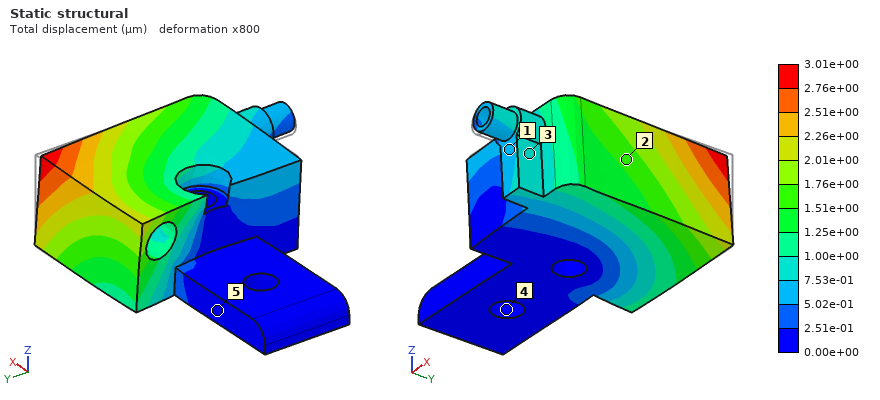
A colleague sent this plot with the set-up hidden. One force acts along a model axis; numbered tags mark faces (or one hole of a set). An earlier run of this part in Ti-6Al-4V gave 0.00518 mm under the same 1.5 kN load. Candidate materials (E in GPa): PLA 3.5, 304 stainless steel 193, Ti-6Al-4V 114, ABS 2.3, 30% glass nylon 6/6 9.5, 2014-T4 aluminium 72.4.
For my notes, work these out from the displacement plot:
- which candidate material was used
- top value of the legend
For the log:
304 stainless steel
3.01e+00 µm
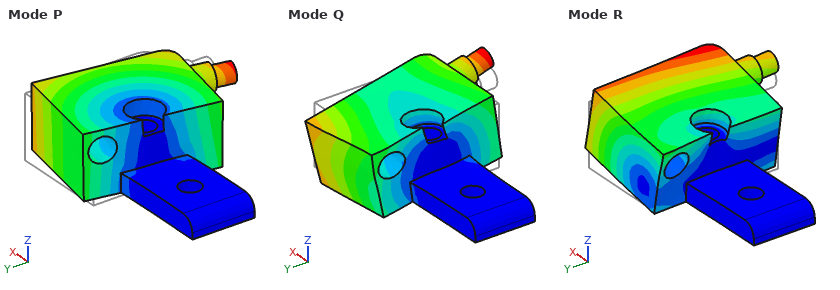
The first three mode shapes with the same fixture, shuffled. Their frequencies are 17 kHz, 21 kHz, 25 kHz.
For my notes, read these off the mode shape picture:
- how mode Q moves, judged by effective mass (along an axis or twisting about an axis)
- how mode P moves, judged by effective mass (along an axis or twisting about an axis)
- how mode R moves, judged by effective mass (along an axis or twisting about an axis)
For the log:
twisting about X
along Y
along Z
